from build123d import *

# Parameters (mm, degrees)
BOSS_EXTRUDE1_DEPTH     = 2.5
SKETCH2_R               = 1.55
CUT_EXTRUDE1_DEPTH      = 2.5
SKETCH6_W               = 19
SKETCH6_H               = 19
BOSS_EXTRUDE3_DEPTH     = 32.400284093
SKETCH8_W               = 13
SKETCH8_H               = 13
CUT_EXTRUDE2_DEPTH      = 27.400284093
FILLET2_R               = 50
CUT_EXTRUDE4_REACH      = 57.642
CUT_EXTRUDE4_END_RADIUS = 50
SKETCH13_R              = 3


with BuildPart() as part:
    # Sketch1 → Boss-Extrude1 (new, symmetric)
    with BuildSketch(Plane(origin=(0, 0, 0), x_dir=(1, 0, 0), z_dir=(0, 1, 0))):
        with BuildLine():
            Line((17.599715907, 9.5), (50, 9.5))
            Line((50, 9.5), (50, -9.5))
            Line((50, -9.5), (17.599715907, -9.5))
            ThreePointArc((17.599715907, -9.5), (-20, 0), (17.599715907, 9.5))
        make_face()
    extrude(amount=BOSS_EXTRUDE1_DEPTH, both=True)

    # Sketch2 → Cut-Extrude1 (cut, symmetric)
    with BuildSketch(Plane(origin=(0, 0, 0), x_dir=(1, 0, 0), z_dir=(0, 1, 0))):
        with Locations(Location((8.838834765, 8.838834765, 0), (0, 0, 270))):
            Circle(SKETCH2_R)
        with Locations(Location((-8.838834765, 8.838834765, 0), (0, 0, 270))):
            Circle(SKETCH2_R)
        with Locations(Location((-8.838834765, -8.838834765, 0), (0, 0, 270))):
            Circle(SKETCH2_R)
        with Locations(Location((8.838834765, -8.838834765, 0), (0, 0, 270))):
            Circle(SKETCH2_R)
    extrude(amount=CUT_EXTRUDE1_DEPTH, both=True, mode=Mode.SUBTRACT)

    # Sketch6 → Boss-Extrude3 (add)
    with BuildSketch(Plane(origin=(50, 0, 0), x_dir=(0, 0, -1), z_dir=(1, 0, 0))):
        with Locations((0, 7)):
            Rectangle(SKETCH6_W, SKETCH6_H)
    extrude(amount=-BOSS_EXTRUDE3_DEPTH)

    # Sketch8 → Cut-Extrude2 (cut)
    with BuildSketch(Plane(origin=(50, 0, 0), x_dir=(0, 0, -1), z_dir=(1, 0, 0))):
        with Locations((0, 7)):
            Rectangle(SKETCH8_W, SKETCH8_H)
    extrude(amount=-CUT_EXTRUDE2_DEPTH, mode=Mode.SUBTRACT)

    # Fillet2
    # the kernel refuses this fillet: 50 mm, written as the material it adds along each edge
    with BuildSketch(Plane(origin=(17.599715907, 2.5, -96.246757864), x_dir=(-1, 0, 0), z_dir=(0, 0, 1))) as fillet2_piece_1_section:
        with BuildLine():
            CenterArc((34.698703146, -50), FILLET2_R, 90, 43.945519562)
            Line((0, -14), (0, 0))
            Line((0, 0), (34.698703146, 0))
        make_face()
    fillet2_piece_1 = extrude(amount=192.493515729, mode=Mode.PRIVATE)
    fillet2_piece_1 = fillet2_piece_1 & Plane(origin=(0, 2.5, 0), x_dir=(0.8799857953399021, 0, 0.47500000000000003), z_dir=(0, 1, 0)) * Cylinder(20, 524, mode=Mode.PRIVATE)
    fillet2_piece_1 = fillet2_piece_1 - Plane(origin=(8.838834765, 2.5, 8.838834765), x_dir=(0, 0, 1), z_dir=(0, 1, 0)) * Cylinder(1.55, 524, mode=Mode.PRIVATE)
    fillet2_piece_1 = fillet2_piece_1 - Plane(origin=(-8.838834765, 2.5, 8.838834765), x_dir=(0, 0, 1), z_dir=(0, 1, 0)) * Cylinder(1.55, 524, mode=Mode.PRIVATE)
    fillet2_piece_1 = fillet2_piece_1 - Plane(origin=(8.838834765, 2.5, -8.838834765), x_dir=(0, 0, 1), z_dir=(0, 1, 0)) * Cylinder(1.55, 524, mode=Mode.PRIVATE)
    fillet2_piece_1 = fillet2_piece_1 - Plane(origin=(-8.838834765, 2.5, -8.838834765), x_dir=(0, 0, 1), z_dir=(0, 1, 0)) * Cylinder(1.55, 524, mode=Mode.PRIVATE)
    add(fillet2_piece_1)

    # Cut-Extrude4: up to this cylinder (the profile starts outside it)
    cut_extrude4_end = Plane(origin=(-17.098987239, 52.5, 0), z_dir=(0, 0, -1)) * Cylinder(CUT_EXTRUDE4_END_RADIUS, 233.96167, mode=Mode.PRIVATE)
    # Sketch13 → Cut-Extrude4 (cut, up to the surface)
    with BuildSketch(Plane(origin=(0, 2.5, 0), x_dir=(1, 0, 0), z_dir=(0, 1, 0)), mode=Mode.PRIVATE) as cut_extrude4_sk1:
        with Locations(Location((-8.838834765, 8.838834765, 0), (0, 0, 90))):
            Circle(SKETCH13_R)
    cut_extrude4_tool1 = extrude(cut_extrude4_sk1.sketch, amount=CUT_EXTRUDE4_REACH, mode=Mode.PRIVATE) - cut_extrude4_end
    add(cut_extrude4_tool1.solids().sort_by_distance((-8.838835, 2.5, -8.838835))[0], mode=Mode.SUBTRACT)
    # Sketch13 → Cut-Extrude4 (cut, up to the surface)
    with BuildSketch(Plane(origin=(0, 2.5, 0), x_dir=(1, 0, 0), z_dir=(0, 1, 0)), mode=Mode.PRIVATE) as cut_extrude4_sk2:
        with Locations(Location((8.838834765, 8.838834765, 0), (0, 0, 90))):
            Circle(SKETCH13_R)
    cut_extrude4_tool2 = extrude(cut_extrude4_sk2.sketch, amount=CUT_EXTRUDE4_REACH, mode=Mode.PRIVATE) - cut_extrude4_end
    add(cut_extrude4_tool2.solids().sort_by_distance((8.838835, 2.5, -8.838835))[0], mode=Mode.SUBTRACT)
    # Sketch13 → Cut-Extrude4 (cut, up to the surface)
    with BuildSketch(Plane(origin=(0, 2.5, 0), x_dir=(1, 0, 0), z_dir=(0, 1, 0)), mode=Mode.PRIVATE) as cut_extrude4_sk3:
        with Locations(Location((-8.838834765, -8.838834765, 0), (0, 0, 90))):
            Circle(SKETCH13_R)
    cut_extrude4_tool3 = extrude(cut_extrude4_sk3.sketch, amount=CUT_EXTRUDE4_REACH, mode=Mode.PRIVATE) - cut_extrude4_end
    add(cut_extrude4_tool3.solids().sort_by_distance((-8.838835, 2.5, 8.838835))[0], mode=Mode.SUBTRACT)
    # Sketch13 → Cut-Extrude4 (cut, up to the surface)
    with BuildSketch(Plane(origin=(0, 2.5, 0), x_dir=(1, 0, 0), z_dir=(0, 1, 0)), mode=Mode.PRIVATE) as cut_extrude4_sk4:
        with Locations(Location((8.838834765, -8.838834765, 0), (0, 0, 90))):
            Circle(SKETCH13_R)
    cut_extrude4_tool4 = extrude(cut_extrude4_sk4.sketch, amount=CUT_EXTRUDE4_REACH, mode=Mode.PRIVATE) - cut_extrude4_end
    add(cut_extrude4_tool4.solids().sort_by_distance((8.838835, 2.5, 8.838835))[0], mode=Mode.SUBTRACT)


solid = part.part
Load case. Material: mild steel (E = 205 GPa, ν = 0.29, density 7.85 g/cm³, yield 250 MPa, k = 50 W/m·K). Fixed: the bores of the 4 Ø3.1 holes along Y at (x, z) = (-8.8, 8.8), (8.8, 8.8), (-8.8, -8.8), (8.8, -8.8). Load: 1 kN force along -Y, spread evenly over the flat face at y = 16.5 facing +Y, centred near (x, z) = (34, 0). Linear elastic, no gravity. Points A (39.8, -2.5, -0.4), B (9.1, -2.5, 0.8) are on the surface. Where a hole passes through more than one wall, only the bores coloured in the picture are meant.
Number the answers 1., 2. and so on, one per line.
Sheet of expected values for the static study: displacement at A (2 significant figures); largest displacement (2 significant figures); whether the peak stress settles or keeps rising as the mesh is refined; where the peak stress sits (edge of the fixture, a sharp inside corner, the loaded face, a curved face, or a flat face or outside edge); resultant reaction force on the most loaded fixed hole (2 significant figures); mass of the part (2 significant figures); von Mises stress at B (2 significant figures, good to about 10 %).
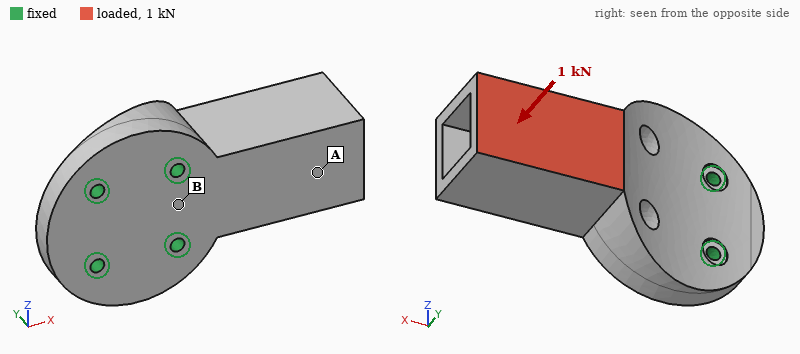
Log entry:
1. 18 µm
2. 28 µm
3. keeps rising
4. edge of the fixture
5. 1.2 kN
6. 140 g
7. 27 MPa
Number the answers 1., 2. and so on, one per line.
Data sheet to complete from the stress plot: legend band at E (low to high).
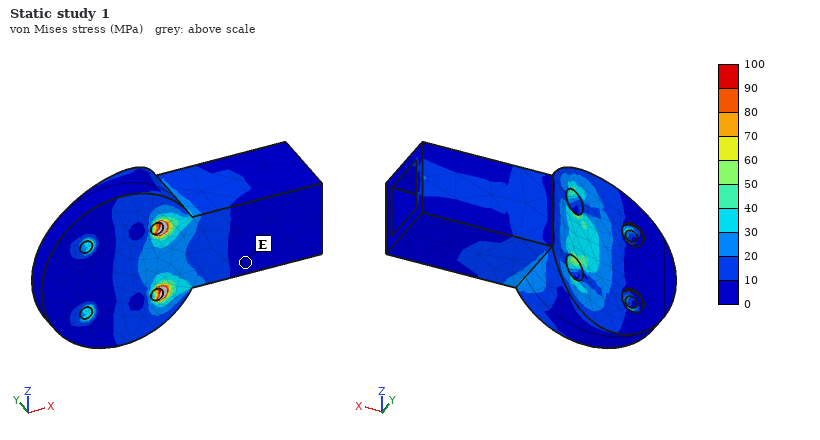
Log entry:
1. 0 to 10 MPa
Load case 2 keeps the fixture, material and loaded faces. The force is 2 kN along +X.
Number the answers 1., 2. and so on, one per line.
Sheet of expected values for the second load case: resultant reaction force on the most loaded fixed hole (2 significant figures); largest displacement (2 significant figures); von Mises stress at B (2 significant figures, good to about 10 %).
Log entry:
1. 1.1 kN
2. 33 µm
3. 29 MPa
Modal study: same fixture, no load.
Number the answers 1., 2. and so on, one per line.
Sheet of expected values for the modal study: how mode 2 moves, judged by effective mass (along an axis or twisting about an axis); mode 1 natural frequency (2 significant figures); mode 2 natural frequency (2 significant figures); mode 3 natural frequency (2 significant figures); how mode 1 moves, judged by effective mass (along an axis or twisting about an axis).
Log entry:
1. along Z
2. 5100 Hz
3. 8900 Hz
4. 16 kHz
5. along Y
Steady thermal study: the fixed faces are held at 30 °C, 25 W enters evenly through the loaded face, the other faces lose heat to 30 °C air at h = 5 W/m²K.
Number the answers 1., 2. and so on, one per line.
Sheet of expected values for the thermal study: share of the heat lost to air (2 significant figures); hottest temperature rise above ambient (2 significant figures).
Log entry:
1. 3.8 %
2. 74 K
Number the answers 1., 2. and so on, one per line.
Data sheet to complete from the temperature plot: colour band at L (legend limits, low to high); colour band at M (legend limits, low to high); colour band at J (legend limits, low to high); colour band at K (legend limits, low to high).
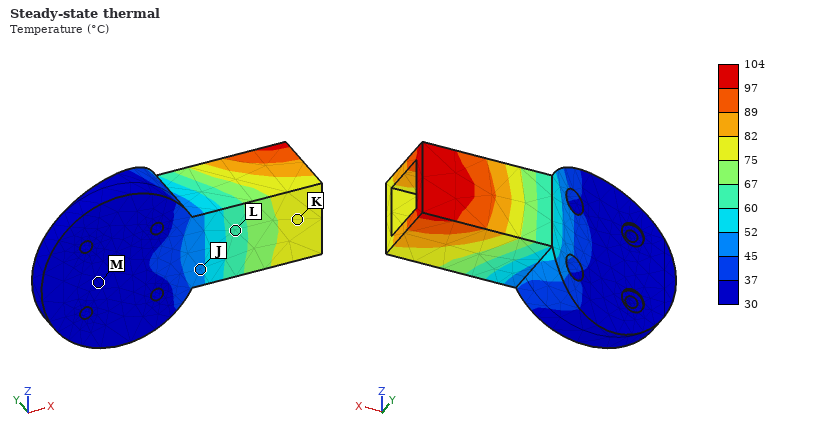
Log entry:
1. 60 to 67 °C
2. 30 to 37 °C
3. 45 to 52 °C
4. 75 to 82 °C
